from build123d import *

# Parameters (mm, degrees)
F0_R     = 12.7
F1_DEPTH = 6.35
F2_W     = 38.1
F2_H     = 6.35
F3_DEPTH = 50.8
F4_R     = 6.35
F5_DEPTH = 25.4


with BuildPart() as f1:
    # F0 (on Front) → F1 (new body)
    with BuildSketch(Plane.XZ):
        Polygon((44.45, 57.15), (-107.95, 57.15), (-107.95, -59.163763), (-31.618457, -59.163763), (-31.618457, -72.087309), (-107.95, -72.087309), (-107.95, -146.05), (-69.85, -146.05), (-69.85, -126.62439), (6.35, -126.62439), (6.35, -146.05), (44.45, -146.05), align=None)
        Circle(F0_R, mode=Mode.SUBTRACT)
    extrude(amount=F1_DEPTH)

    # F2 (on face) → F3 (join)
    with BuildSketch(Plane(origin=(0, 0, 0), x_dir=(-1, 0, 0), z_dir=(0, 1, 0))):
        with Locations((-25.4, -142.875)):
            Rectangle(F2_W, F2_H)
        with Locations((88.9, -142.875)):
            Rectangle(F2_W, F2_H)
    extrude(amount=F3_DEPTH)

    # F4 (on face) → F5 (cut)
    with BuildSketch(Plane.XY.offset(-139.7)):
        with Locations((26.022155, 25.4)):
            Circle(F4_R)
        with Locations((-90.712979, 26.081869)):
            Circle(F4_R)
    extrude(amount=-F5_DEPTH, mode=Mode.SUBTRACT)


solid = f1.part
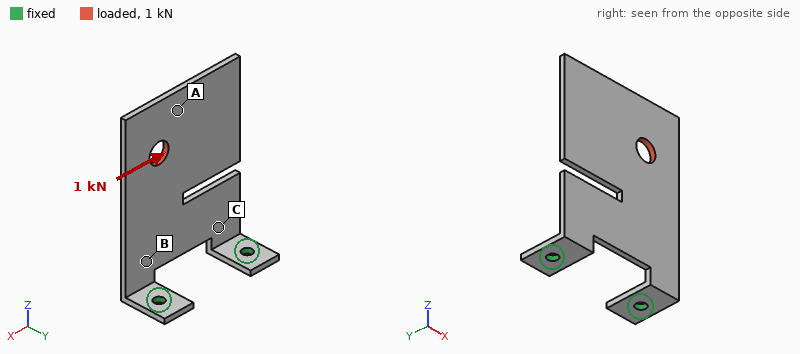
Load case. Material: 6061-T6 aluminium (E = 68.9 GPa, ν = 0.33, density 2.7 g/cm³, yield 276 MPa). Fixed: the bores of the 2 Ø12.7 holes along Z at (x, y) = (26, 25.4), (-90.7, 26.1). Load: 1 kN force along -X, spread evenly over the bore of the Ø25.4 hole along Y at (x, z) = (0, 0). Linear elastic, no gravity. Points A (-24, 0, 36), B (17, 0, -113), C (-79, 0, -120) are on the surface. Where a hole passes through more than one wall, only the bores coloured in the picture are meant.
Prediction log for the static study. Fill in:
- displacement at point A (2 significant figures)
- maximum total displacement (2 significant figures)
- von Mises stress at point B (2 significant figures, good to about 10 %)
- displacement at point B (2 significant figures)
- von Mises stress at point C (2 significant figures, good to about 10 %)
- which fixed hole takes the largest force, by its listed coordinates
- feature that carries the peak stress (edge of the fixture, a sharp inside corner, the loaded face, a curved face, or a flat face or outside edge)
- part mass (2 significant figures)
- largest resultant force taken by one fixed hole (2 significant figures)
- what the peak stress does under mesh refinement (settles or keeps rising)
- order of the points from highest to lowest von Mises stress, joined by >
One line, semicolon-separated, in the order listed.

0.34 mm; 0.48 mm; 15 MPa; 0.11 mm; 24 MPa; (-90.7, 26.1); edge of the fixture; 540 g; 1.4 kN; keeps rising; C > B > A
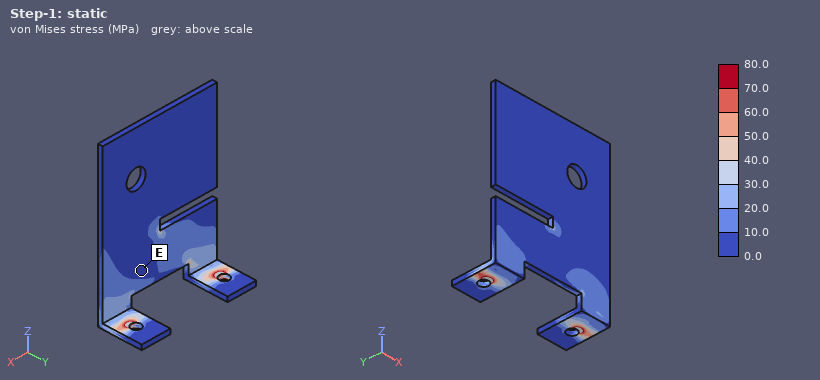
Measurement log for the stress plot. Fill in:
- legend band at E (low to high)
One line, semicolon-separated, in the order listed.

0.0 to 10.0 MPa
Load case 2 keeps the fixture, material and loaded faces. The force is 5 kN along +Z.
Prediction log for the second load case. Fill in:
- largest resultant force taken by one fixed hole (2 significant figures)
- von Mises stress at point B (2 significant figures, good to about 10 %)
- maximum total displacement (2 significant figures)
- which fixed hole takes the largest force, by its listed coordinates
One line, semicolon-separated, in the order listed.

3.8 kN; 29 MPa; 3.1 mm; (26, 25.4)
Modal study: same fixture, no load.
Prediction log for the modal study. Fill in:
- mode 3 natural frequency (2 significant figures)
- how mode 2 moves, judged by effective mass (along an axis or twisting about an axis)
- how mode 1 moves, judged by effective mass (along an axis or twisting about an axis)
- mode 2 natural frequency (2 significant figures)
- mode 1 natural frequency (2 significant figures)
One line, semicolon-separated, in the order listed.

510 Hz; twisting about Z; along Y; 260 Hz; 77 Hz
